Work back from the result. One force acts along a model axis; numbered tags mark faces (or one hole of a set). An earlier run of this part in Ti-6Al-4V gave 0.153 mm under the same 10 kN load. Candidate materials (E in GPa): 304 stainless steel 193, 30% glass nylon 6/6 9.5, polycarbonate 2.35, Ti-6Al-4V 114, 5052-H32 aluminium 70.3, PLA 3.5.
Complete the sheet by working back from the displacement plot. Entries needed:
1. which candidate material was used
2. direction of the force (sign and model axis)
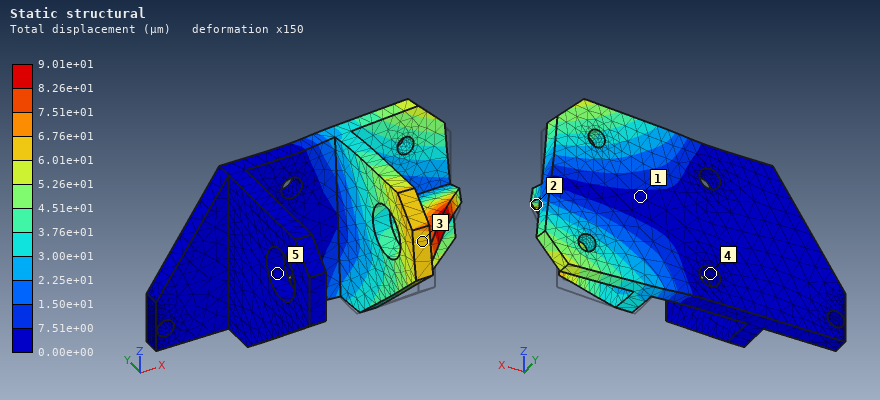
304 stainless steel
+Z
